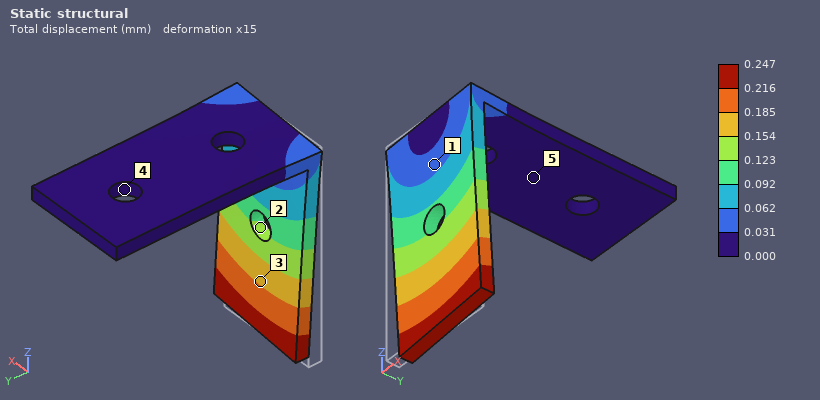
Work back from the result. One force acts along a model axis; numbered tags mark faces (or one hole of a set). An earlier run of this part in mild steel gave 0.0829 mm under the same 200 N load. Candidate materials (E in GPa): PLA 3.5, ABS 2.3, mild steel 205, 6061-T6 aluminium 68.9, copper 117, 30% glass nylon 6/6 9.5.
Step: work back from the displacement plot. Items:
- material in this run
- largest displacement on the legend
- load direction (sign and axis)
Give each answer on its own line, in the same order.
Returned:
6061-T6 aluminium
0.247 mm
+X
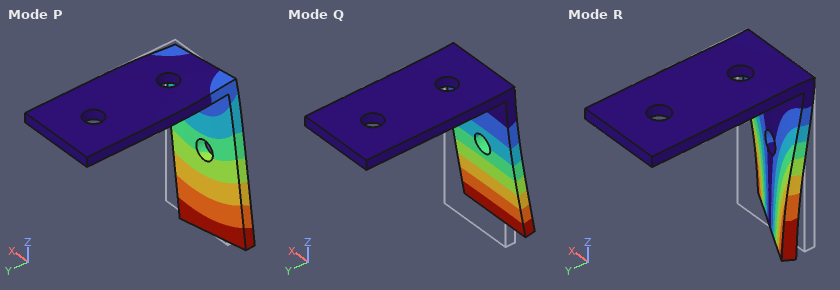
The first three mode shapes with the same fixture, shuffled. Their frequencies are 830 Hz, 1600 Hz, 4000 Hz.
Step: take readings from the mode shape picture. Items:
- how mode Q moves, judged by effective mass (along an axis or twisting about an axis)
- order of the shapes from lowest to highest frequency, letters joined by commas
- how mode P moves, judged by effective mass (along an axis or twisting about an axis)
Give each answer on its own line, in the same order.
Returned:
along Y
Q, P, R
along X
